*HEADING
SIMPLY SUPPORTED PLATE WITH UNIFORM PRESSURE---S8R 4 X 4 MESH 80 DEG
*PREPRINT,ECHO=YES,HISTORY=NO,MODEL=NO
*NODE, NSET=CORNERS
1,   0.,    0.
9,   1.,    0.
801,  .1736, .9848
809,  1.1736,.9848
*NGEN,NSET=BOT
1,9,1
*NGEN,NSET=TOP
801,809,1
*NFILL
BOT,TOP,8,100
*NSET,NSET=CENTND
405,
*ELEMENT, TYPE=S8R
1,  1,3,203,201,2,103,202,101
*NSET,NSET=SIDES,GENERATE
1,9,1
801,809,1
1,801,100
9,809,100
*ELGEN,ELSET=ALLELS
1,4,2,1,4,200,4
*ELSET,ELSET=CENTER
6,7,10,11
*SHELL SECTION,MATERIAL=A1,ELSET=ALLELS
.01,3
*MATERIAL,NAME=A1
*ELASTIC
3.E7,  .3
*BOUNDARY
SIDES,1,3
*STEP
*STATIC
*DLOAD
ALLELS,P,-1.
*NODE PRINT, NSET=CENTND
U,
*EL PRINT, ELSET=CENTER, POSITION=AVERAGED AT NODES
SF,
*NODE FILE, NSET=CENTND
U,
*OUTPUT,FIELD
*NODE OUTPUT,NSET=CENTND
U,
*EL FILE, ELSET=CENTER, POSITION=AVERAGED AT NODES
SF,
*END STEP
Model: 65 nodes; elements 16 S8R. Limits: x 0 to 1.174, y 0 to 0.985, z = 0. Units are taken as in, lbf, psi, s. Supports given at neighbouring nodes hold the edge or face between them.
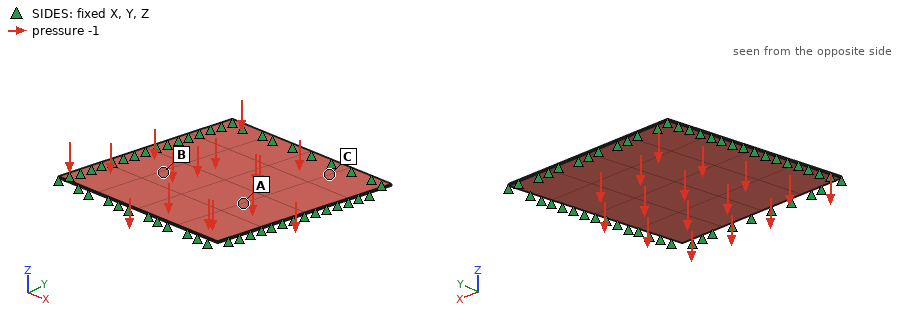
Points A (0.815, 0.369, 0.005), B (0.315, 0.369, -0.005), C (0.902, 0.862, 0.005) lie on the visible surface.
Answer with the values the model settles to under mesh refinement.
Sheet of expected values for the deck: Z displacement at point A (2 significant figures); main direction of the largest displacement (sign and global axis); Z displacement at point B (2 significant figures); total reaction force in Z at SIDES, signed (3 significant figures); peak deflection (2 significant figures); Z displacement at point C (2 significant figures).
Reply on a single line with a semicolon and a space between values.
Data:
-9.8e-04 in; -Z; -9.2e-04 in; 0.985 lbf; 0.0014 in; -3.7e-04 in
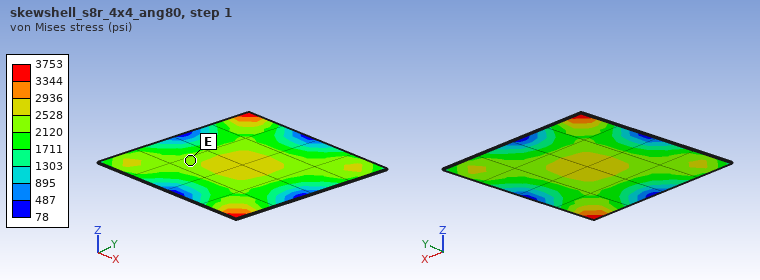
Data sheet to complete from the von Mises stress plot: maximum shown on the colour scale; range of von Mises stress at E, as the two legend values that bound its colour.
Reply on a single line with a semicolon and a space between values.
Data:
3753 psi; 2120 to 2528 psi
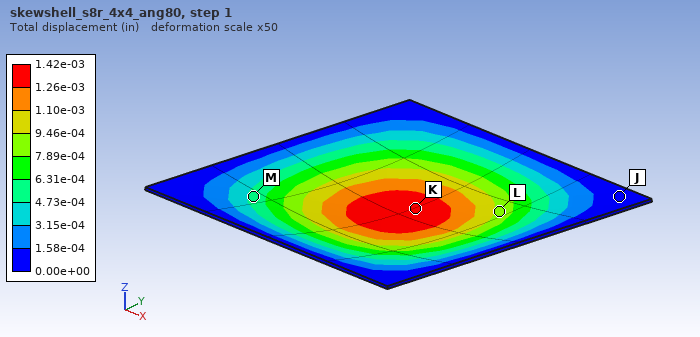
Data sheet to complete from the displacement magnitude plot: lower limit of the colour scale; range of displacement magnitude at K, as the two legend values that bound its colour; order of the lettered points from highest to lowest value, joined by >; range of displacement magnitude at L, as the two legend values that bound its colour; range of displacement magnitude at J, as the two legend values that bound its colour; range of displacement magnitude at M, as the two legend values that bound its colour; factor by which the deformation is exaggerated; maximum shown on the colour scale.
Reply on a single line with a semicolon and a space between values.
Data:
0.00e+00 in; 1.26e-03 to 1.42e-03 in; K > L > M > J; 7.89e-04 to 9.46e-04 in; 0.00e+00 to 1.58e-04 in; 4.73e-04 to 6.31e-04 in; 50; 1.42e-03 in
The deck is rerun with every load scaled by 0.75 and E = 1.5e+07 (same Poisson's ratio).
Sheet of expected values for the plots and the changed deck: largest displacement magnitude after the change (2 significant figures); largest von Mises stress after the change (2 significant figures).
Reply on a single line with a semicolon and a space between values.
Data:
0.0021 in; 2800 psi
